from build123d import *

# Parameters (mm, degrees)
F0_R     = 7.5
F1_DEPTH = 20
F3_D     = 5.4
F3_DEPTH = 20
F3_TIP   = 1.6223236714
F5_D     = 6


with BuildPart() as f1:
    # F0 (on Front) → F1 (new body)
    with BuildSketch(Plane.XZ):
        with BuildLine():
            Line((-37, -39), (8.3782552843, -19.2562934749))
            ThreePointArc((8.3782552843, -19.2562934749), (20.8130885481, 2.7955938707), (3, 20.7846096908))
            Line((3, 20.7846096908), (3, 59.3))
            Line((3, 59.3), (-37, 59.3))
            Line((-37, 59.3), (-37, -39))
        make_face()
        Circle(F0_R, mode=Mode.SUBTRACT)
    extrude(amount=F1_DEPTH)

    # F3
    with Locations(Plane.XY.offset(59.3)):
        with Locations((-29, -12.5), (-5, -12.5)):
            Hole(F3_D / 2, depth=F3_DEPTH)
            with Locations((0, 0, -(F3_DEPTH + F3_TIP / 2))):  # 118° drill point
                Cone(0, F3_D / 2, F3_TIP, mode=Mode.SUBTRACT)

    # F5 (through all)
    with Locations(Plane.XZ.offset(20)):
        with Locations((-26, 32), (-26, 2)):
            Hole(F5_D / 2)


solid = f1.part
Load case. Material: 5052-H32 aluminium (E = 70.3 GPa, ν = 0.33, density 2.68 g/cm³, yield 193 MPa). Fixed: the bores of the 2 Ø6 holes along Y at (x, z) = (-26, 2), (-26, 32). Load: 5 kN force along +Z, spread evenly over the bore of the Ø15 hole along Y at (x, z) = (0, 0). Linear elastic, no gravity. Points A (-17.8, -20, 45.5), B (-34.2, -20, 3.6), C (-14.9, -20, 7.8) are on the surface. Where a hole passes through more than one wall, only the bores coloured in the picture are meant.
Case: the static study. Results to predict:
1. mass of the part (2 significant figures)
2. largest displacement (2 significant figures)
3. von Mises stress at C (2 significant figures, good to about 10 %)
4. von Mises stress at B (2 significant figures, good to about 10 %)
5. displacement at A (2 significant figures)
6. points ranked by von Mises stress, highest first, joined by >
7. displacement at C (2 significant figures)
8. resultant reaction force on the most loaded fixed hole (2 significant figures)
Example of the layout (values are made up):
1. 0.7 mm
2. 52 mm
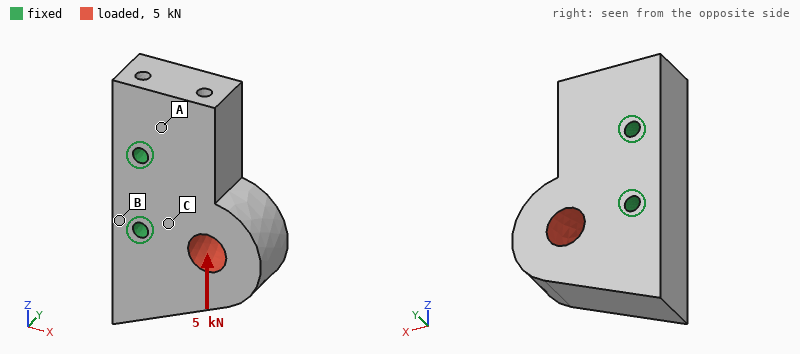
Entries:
1. 210 g
2. 16 µm
3. 15 MPa
4. 7.8 MPa
5. 4.2 µm
6. C > B > A
7. 3.4 µm
8. 4.4 kN
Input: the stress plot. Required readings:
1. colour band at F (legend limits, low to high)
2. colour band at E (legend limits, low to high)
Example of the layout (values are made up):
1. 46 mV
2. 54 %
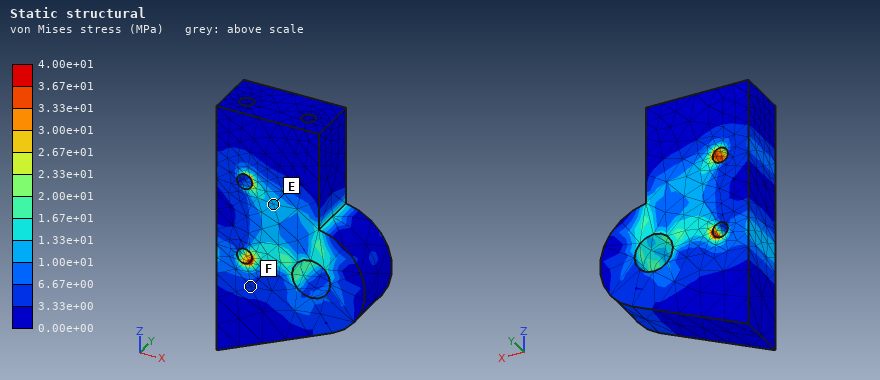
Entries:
1. 3.33e+00 to 6.67e+00 MPa
2. 1.00e+01 to 1.33e+01 MPa
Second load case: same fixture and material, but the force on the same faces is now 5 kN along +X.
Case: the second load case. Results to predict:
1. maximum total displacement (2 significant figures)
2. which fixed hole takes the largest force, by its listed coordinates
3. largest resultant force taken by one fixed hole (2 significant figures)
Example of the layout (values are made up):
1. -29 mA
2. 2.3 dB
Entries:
1. 10 µm
2. (-26, 2)
3. 5.0 kN
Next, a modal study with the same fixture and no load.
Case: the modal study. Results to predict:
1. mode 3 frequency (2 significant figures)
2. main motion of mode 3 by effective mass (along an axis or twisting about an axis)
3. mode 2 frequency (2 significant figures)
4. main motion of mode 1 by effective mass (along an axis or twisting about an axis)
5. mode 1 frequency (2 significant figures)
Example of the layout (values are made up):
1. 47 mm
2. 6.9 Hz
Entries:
1. 9700 Hz
2. twisting about X
3. 8600 Hz
4. along Y
5. 7100 Hz
